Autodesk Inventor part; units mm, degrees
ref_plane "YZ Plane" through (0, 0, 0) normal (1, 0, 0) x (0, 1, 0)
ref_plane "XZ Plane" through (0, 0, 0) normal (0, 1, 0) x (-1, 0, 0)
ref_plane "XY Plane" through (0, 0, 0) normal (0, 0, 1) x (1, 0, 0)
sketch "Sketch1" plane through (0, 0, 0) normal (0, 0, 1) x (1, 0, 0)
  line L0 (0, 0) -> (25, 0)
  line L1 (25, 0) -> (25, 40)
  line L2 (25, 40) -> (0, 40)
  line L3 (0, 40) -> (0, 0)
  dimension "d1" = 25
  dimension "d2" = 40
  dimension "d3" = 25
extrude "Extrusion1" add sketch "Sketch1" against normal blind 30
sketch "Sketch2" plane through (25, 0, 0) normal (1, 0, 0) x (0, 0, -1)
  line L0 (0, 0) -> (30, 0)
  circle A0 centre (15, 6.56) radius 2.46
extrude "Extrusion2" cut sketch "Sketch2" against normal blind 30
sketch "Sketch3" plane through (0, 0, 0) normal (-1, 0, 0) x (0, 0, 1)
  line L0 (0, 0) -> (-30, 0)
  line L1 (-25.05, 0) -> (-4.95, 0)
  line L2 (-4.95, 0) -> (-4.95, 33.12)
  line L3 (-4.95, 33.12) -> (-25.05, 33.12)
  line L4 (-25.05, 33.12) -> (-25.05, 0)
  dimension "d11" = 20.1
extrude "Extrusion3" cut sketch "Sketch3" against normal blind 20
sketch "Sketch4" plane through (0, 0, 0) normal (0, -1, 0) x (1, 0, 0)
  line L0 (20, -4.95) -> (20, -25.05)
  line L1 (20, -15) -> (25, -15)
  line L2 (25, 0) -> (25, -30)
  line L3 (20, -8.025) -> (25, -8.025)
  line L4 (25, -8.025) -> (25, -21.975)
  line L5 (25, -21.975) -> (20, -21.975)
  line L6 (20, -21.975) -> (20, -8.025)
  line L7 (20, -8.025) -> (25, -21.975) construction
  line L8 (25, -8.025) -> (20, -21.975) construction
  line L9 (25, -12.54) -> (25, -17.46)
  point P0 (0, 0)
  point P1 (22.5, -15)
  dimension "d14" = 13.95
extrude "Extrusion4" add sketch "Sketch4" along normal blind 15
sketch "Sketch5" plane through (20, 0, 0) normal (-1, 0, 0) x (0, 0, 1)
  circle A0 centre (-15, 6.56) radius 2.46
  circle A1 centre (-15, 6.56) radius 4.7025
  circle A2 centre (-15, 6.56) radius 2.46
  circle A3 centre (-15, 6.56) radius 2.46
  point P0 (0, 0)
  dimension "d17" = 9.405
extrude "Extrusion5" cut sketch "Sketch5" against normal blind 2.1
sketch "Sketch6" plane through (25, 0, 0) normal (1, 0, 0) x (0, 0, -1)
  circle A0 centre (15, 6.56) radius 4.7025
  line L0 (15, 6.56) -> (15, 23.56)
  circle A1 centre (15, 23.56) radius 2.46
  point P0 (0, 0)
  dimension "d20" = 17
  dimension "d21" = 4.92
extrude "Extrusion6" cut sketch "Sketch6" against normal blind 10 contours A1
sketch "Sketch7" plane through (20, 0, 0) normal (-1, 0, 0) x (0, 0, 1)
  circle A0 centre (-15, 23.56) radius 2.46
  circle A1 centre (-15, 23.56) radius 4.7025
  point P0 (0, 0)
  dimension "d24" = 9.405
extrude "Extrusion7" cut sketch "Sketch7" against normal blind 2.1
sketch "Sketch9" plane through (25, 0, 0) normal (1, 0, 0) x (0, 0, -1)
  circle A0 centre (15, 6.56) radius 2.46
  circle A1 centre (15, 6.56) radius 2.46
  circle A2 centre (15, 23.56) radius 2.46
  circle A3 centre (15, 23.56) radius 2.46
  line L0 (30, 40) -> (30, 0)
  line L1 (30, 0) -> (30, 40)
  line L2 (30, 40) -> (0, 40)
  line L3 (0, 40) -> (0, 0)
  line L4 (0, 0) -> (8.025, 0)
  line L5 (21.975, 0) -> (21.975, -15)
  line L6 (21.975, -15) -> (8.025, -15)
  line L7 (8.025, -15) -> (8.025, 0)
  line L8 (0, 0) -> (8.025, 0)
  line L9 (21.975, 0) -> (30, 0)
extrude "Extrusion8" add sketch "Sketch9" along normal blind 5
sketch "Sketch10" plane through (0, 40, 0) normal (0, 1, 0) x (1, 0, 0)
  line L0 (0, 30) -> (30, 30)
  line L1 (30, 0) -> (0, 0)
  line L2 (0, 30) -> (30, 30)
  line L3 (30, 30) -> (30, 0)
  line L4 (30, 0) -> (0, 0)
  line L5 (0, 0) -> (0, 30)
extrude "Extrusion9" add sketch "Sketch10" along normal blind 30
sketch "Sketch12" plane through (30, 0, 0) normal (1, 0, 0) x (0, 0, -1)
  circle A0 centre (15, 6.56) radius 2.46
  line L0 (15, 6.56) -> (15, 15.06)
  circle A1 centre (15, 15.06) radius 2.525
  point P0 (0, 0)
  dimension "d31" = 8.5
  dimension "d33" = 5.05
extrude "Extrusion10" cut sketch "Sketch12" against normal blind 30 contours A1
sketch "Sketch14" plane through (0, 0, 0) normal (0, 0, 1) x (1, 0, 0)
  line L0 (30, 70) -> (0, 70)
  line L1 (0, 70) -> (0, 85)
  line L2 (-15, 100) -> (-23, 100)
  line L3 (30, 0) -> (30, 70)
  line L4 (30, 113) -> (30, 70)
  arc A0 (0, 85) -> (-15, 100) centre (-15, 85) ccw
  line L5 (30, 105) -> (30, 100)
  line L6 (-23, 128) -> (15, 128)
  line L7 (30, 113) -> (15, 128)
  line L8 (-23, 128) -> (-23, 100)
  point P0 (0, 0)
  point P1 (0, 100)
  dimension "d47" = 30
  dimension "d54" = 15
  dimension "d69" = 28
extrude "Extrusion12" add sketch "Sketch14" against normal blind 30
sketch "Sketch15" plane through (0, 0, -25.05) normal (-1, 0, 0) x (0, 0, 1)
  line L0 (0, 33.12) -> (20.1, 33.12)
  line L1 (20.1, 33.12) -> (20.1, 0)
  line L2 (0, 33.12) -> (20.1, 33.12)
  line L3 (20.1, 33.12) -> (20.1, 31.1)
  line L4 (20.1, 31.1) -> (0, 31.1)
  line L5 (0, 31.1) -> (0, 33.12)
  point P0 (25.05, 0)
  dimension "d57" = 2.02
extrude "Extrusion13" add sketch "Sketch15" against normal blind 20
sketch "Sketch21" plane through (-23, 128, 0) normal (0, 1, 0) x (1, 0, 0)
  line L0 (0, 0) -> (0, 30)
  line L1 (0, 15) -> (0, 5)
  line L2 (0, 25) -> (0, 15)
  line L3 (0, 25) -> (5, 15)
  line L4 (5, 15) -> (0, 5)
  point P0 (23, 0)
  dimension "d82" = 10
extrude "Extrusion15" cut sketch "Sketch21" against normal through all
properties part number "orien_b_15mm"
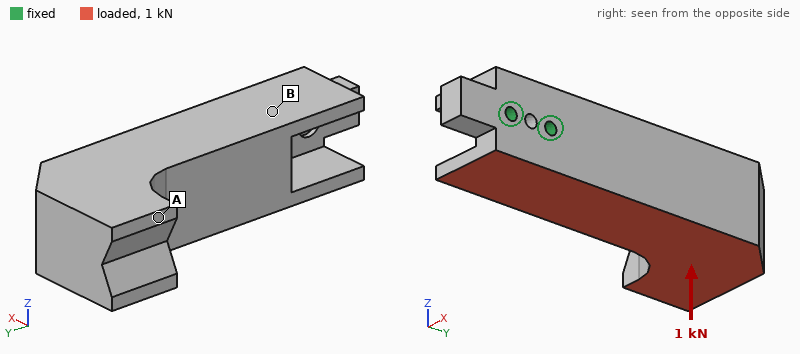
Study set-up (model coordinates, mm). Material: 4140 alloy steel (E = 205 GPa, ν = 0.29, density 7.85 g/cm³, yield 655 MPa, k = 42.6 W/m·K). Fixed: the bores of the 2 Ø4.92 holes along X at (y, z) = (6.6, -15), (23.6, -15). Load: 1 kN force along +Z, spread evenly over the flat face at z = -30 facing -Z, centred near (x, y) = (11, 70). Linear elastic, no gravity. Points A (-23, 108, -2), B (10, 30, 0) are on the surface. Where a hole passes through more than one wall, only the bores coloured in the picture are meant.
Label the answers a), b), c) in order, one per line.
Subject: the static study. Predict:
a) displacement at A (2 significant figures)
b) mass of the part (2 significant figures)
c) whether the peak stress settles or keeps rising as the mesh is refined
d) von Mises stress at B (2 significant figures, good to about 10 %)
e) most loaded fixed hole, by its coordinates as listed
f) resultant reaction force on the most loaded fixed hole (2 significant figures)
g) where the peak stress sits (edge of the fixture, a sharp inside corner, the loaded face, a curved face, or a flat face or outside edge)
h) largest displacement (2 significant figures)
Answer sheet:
a) 34 µm
b) 940 g
c) keeps rising
d) 12 MPa
e) (23.6, -15)
f) 3.0 kN
g) edge of the fixture
h) 41 µm
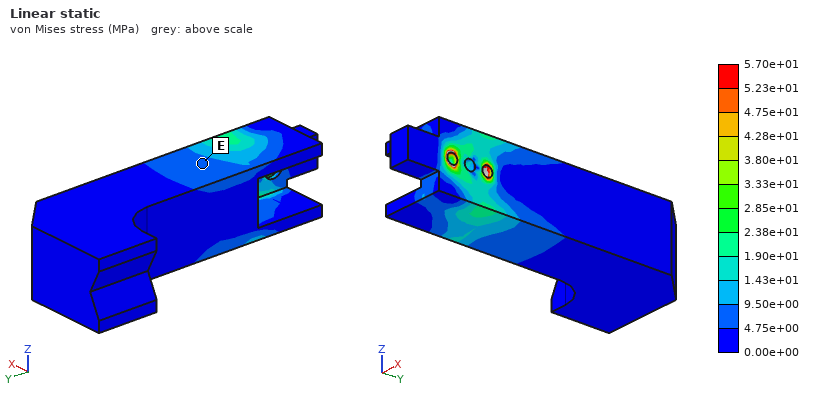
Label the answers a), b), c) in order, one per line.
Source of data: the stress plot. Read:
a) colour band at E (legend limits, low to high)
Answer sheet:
a) 4.75e+00 to 9.50e+00 MPa
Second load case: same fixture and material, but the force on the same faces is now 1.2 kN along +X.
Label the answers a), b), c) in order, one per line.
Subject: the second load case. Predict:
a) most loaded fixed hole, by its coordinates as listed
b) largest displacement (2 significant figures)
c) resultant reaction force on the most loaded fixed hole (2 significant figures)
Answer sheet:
a) (23.6, -15)
b) 66 µm
c) 3.3 kN
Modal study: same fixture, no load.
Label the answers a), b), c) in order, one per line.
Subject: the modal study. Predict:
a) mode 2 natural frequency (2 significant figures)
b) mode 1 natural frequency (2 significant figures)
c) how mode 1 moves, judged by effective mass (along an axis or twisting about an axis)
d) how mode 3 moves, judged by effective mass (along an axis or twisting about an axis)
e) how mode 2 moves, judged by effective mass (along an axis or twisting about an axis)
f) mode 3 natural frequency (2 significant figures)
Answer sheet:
a) 990 Hz
b) 840 Hz
c) along X
d) twisting about Y
e) along Z
f) 2700 Hz
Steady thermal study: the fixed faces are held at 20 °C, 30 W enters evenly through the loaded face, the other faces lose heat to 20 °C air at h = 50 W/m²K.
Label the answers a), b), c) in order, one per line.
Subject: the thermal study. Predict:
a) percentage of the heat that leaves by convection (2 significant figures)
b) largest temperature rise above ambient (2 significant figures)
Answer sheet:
a) 47 %
b) 28 K
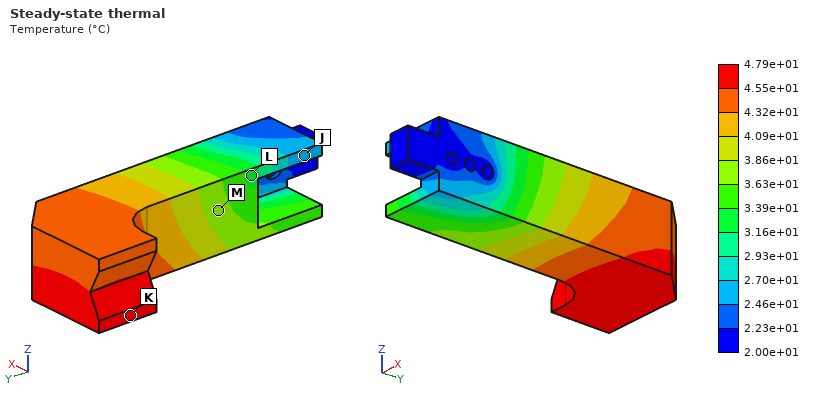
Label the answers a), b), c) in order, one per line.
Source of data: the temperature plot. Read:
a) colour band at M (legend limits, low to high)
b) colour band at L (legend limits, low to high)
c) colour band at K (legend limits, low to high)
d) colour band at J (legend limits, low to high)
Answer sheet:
a) 3.63e+01 to 3.86e+01 °C
b) 3.16e+01 to 3.39e+01 °C
c) 4.55e+01 to 4.79e+01 °C
d) 2.46e+01 to 2.70e+01 °C
